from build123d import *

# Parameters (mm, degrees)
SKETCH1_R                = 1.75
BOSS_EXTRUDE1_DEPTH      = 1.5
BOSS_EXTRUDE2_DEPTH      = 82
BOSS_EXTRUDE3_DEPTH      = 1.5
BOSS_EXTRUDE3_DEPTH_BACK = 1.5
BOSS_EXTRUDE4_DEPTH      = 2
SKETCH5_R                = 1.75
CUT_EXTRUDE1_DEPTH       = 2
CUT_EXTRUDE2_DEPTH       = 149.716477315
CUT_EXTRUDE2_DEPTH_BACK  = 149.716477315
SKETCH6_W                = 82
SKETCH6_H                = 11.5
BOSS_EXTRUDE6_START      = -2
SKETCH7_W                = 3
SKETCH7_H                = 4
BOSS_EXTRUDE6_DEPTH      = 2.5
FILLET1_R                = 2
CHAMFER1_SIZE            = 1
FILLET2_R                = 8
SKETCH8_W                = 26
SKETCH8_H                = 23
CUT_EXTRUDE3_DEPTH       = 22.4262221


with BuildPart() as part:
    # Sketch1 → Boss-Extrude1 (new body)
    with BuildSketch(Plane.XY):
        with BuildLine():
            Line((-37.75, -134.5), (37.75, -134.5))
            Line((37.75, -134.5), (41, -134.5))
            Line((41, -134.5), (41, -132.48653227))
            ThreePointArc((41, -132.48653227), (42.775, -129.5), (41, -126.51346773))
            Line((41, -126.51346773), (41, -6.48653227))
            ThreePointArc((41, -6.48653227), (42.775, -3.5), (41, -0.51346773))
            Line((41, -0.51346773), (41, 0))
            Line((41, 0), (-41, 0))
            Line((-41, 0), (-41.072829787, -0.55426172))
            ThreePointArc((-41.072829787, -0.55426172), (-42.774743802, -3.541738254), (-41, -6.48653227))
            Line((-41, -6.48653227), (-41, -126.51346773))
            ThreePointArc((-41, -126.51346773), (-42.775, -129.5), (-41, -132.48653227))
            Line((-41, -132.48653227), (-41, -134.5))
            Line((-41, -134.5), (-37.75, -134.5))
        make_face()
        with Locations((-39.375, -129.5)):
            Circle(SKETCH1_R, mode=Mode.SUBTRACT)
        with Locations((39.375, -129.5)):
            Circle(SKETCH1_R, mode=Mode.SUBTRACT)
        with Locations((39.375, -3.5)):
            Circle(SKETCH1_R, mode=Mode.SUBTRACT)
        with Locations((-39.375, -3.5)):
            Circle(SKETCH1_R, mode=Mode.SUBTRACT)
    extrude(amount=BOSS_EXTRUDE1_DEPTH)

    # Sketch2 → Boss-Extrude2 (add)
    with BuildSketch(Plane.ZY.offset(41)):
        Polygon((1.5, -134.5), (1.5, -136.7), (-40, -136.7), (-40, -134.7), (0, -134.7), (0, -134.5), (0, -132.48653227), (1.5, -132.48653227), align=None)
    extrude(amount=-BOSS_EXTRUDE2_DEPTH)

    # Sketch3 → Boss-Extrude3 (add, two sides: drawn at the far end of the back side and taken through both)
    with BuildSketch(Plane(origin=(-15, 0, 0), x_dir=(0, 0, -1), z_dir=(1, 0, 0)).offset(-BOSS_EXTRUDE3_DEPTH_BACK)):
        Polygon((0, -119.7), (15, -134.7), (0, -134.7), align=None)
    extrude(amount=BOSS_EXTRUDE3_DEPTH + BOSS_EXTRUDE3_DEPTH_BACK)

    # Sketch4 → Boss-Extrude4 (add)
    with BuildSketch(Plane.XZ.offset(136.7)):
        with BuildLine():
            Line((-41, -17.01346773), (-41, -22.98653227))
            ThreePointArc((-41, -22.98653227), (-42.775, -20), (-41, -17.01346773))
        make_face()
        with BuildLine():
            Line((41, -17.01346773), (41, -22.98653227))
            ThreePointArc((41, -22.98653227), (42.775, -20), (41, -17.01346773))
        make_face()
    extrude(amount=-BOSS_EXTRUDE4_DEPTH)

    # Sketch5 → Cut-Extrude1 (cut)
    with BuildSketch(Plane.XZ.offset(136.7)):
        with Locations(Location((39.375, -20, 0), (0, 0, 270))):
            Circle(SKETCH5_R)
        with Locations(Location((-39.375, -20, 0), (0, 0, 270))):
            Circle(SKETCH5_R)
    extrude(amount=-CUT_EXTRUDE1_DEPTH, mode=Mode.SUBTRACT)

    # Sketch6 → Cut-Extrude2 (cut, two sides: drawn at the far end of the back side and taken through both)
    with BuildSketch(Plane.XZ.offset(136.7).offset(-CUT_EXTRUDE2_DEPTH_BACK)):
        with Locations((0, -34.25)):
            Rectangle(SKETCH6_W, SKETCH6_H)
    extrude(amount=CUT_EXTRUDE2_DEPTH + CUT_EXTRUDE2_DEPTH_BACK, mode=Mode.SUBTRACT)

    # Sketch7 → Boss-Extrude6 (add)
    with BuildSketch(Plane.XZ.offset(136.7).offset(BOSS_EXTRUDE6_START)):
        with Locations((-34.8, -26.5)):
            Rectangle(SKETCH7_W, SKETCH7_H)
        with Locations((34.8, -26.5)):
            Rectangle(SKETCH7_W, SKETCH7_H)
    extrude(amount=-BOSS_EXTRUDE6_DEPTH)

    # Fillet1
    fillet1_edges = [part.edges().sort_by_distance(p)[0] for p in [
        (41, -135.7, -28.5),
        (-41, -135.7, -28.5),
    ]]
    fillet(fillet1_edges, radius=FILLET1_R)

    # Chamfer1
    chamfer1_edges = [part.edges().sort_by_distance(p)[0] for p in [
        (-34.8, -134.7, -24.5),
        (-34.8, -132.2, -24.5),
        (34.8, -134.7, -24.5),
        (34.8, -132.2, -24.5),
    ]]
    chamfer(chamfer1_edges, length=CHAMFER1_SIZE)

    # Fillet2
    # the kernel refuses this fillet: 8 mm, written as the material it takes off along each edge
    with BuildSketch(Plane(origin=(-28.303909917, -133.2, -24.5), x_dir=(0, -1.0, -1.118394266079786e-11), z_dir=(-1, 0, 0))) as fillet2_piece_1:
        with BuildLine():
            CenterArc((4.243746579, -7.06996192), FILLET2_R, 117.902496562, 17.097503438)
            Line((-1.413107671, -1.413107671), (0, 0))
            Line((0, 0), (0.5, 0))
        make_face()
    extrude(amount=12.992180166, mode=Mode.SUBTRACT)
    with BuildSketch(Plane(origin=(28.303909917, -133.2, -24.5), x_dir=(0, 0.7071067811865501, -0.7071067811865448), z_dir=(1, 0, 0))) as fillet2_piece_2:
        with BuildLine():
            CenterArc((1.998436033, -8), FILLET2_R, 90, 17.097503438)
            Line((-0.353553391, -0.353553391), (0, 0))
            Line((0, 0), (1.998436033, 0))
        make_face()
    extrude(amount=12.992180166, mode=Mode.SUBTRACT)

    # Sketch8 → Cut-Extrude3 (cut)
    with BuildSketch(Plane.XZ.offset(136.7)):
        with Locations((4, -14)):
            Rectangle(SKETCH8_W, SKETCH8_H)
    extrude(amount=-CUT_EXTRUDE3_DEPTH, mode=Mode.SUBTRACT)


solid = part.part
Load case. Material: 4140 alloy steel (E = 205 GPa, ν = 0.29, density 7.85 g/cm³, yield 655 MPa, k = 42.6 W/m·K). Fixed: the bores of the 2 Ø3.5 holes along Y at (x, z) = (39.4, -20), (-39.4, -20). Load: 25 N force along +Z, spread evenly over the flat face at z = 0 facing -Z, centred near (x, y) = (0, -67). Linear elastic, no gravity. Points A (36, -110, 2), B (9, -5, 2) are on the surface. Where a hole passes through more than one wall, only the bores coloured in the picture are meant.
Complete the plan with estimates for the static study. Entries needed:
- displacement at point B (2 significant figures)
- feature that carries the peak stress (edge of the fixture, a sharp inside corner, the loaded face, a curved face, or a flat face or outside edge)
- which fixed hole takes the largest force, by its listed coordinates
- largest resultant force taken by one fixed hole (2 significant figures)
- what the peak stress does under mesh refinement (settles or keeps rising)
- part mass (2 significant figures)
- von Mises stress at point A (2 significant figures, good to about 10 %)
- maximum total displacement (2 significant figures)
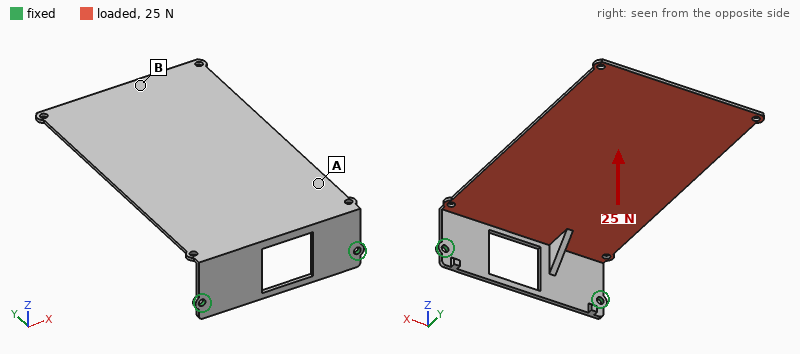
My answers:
1.8 mm
edge of the fixture
(-39.4, -20)
18 N
keeps rising
160 g
30 MPa
1.9 mm
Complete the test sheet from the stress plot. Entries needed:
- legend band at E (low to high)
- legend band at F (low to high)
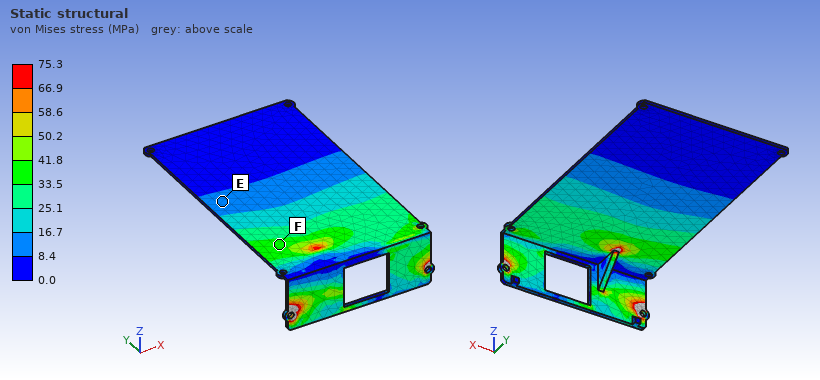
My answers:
8.4 to 16.7 MPa
33.5 to 41.8 MPa
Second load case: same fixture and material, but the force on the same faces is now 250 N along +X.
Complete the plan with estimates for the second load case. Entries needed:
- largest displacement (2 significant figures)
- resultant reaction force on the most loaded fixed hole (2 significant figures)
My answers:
0.97 mm
270 N
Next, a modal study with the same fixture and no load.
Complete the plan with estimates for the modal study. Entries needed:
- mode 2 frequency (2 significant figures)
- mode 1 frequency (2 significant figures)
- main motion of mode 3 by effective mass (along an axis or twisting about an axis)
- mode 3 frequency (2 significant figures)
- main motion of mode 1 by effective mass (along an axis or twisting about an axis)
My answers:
240 Hz
63 Hz
along X
320 Hz
along Z
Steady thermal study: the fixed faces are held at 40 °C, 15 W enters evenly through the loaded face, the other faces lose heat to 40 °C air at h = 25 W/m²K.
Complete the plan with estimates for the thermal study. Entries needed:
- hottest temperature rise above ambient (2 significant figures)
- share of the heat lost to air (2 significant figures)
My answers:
47 K
85 %
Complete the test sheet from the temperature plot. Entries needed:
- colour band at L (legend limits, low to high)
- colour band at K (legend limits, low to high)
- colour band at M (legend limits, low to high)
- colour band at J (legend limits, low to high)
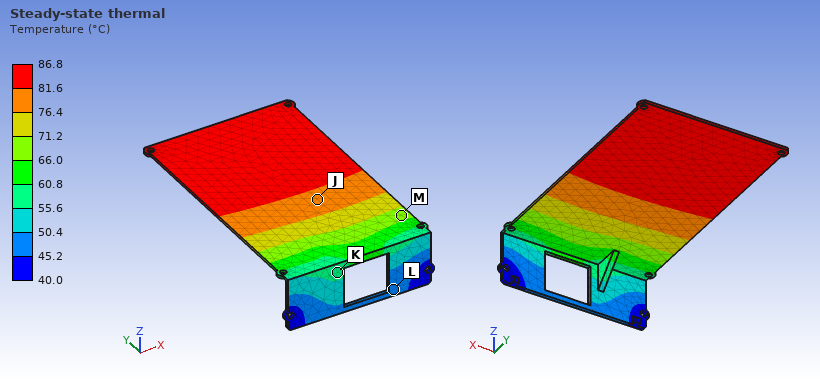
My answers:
45.2 to 50.4 °C
55.6 to 60.8 °C
66.0 to 71.2 °C
76.4 to 81.6 °C
